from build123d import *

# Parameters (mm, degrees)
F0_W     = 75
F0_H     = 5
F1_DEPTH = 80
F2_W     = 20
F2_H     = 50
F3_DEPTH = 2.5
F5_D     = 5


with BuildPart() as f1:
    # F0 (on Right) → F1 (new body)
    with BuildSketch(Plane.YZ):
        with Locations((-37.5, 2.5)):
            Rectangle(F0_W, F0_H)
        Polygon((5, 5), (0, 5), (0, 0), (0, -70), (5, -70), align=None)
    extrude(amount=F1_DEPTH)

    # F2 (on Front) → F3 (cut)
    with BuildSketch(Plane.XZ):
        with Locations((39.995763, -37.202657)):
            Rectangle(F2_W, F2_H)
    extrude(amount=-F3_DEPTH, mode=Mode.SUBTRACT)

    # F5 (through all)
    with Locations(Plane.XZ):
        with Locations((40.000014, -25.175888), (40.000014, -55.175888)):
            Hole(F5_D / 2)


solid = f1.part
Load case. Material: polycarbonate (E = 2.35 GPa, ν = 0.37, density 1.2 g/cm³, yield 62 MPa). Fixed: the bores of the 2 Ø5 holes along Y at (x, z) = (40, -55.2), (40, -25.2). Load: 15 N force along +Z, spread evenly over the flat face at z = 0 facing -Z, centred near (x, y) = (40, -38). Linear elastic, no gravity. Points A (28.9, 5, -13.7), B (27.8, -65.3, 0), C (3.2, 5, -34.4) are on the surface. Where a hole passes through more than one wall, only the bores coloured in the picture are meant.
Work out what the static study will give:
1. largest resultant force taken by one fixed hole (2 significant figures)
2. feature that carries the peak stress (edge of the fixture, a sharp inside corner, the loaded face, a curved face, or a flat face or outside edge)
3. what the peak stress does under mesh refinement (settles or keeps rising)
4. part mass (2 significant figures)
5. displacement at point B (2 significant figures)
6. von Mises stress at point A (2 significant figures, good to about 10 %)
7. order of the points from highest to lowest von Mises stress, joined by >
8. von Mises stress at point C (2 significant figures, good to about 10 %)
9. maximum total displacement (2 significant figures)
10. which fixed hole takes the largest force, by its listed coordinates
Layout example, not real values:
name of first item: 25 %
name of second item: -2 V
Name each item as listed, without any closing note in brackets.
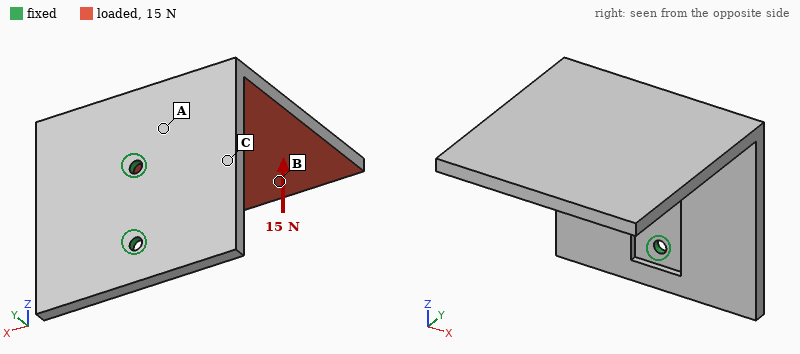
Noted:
largest resultant force taken by one fixed hole: 27 N
feature that carries the peak stress: edge of the fixture
what the peak stress does under mesh refinement: keeps rising
part mass: 69 g
displacement at point B: 1.3 mm
von Mises stress at point A: 2.1 MPa
order of the points from highest to lowest von Mises stress, joined by >: A > C > B
von Mises stress at point C: 1.1 MPa
maximum total displacement: 1.5 mm
which fixed hole takes the largest force, by its listed coordinates: (40, -55.2)
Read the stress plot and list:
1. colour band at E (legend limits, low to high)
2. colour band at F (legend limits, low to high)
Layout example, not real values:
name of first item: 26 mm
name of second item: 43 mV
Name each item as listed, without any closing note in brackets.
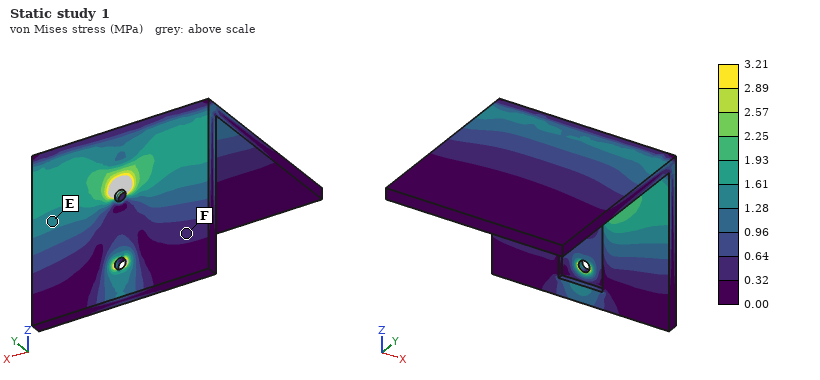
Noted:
colour band at E: 1.28 to 1.61 MPa
colour band at F: 0.32 to 0.64 MPa
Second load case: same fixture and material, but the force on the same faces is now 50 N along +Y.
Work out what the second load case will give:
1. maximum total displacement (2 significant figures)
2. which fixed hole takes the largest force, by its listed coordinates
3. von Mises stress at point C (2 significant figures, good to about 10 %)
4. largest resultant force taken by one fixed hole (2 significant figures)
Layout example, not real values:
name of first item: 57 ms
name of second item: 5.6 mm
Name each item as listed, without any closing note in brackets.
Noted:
maximum total displacement: 1.5 mm
which fixed hole takes the largest force, by its listed coordinates: (40, -25.2)
von Mises stress at point C: 1.7 MPa
largest resultant force taken by one fixed hole: 87 N
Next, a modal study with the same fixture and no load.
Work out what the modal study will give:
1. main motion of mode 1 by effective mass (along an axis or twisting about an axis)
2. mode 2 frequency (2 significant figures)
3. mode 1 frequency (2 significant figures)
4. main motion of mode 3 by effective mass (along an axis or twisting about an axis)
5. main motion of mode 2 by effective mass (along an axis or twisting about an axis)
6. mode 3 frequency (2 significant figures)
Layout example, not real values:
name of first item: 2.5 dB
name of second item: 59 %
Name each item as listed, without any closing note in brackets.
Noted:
main motion of mode 1 by effective mass: along X
mode 2 frequency: 99 Hz
mode 1 frequency: 93 Hz
main motion of mode 3 by effective mass: along Y
main motion of mode 2 by effective mass: along Z
mode 3 frequency: 330 Hz
